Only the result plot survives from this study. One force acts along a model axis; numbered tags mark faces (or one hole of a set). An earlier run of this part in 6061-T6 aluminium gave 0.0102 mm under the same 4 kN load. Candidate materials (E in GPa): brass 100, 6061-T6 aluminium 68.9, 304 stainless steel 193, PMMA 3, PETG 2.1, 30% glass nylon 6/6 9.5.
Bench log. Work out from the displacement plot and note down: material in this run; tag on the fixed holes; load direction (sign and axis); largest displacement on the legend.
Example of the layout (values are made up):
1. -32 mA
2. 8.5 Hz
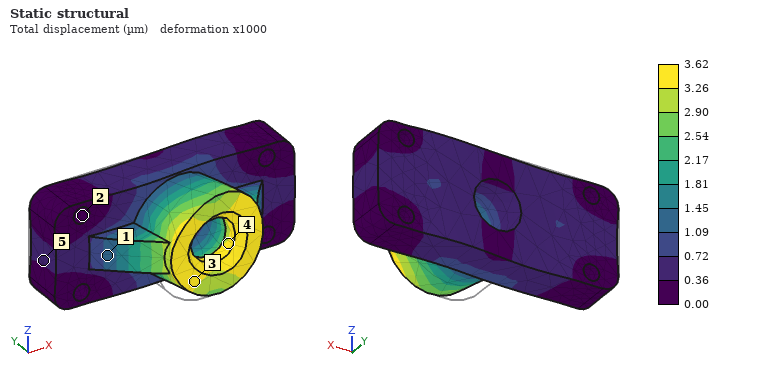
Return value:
1. 304 stainless steel
2. 2
3. +X
4. 3.62 µm
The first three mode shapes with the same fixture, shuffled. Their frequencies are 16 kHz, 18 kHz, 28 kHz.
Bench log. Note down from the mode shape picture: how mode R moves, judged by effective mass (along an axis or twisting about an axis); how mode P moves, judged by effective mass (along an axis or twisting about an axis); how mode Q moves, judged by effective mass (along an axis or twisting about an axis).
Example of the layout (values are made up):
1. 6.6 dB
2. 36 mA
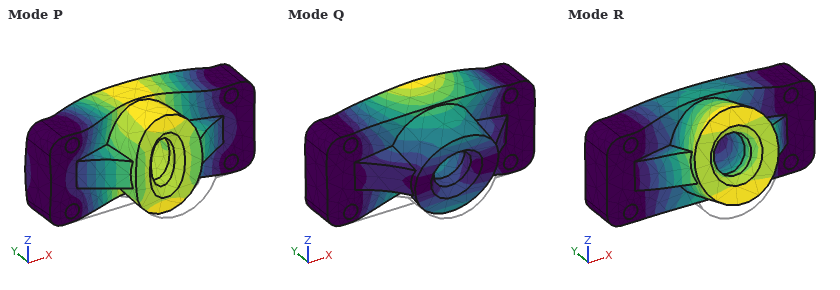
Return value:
1. along Z
2. along Y
3. along Z
